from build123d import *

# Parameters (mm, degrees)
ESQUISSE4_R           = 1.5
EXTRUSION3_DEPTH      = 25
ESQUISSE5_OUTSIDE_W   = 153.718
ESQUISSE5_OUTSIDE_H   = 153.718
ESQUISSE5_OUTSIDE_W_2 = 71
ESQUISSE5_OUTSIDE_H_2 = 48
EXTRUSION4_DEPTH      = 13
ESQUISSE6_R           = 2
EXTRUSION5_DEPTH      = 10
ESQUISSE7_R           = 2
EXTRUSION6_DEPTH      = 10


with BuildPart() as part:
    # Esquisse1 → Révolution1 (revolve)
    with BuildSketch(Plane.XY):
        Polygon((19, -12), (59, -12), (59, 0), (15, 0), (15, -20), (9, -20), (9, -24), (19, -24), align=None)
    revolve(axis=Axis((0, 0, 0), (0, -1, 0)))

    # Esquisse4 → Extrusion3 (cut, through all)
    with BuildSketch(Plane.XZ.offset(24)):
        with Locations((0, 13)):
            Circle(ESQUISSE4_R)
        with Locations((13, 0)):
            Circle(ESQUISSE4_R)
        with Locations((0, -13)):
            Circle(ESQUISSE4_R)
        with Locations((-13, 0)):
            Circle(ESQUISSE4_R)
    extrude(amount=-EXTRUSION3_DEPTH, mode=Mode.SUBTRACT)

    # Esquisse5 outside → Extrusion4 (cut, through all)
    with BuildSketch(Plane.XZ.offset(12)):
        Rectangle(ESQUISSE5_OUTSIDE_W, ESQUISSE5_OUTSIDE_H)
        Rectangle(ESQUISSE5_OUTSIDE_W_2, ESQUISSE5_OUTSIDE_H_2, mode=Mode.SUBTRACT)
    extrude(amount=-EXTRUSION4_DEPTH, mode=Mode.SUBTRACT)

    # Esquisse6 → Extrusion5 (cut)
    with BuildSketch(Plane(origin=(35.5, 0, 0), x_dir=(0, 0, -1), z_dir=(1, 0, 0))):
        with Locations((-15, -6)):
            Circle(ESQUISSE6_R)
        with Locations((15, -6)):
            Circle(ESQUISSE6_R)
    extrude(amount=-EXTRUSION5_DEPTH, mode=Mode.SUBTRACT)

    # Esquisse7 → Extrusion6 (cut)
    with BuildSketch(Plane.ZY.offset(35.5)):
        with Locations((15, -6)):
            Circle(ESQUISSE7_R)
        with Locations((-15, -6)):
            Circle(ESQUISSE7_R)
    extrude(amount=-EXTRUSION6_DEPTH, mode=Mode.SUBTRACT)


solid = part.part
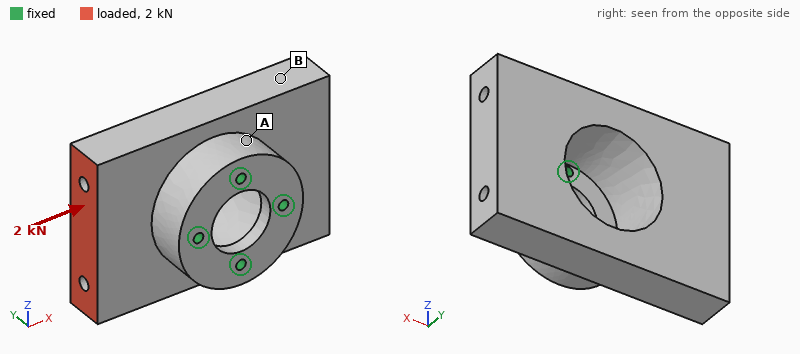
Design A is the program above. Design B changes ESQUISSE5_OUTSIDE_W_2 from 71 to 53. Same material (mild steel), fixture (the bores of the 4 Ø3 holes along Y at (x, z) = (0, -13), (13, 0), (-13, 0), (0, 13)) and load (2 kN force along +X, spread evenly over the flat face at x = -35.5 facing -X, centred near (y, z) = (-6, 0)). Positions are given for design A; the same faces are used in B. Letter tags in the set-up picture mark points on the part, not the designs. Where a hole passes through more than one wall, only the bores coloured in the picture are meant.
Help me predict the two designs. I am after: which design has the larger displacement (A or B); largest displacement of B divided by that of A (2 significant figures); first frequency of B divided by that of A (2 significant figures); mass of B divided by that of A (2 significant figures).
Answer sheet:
A
0.92
1.4
0.74
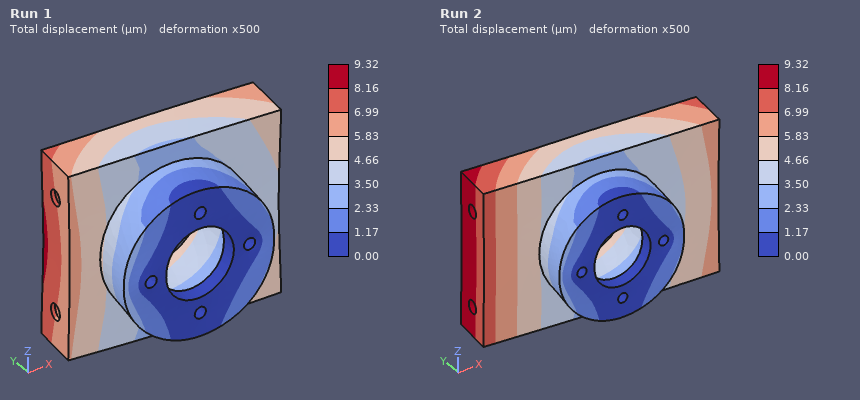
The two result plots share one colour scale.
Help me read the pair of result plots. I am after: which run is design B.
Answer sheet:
Run 1
